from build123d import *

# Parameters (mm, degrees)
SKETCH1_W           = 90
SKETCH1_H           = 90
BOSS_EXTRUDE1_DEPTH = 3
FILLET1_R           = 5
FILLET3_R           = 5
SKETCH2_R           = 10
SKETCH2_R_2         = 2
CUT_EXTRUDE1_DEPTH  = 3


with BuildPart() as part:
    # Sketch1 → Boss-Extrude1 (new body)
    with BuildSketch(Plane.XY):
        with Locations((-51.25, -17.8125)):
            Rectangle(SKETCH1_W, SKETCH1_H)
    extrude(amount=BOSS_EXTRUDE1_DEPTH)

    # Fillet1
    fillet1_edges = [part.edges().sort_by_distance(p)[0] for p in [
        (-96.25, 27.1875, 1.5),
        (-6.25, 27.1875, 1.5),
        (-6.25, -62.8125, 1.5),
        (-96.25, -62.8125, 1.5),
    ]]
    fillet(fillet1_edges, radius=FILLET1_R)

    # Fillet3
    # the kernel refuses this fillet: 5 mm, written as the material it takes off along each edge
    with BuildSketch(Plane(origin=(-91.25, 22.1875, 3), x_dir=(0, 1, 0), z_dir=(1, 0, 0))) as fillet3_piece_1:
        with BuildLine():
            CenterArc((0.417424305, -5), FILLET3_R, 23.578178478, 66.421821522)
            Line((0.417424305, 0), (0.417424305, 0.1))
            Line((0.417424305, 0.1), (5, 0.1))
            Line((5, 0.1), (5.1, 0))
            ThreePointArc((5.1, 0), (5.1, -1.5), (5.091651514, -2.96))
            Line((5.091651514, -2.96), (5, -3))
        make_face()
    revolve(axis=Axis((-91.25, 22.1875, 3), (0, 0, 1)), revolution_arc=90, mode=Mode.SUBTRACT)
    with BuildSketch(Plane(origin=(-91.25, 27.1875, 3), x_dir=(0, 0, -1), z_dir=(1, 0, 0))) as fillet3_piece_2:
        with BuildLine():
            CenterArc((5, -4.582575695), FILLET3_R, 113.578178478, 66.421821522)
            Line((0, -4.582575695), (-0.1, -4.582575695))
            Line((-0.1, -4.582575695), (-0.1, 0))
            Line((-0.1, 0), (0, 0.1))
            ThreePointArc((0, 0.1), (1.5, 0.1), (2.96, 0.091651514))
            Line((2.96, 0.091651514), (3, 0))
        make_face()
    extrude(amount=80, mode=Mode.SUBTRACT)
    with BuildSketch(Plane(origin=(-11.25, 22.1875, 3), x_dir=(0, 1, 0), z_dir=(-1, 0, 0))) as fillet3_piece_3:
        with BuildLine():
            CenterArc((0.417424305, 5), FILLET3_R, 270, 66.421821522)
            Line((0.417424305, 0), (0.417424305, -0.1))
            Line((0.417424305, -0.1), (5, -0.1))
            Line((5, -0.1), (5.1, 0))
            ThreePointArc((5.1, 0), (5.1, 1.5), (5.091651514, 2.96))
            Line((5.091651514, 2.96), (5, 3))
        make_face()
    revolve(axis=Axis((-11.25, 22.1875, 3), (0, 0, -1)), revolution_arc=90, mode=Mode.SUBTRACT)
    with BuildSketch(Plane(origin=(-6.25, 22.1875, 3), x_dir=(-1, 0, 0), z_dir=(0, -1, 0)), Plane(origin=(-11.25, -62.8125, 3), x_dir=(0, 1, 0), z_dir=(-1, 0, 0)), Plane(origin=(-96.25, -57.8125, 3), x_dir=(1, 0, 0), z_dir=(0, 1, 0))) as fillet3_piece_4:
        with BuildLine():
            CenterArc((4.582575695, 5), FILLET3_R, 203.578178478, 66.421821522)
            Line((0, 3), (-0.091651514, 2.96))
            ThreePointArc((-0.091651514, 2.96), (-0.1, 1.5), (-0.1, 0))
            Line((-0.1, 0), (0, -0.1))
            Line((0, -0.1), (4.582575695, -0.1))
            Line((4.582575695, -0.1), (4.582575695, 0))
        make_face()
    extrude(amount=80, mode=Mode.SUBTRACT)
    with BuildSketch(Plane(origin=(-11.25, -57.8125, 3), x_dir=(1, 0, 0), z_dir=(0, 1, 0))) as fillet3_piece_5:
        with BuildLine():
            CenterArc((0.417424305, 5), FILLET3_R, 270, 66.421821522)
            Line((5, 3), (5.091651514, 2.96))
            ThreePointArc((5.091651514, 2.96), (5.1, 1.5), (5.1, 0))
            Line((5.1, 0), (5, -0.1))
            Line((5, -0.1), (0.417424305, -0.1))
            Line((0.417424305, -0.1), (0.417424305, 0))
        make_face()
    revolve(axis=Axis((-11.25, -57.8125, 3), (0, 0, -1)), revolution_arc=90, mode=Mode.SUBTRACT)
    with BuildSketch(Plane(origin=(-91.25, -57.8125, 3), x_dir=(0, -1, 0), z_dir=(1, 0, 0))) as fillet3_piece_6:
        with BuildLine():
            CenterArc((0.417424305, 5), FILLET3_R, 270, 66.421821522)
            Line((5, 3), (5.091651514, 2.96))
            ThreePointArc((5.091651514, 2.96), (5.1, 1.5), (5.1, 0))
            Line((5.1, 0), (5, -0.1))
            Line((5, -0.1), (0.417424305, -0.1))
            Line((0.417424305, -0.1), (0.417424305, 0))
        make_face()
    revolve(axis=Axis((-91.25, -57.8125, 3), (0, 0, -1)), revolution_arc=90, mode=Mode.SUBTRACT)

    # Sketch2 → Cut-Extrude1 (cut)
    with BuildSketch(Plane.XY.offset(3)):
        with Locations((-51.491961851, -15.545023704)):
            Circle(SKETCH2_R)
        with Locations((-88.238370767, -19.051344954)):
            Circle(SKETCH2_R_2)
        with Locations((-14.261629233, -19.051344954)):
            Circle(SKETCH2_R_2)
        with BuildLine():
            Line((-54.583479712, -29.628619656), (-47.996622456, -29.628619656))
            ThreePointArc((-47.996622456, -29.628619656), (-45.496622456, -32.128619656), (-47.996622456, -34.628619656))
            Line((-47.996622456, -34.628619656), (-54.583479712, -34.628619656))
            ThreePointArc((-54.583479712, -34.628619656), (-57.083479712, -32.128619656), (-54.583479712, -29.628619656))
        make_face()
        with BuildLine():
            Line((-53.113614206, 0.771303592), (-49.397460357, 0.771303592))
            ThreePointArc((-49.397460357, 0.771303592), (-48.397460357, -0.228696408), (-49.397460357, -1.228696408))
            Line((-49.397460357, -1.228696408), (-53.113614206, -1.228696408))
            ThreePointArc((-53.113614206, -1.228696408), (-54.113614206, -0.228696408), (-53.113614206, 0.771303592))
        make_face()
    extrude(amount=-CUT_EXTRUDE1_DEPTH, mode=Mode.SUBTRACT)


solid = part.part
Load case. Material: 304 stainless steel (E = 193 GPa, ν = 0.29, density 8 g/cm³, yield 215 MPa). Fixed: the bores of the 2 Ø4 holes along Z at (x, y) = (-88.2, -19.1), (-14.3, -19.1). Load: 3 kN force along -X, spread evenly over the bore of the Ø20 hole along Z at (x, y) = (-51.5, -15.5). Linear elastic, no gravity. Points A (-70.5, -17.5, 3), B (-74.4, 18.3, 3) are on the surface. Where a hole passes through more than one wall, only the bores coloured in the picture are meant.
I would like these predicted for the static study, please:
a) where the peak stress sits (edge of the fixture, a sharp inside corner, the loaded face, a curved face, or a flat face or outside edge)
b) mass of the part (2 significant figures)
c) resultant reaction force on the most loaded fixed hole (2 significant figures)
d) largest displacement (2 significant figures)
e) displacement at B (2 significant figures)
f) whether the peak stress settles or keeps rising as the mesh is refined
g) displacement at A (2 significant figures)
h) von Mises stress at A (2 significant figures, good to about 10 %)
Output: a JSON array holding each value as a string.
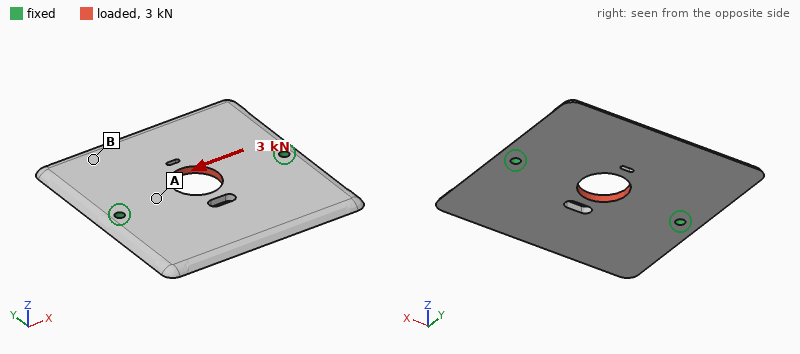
["edge of the fixture", "170 g", "1.5 kN", "4.5 µm", "3.3 µm", "keeps rising", "2.5 µm", "21 MPa"]
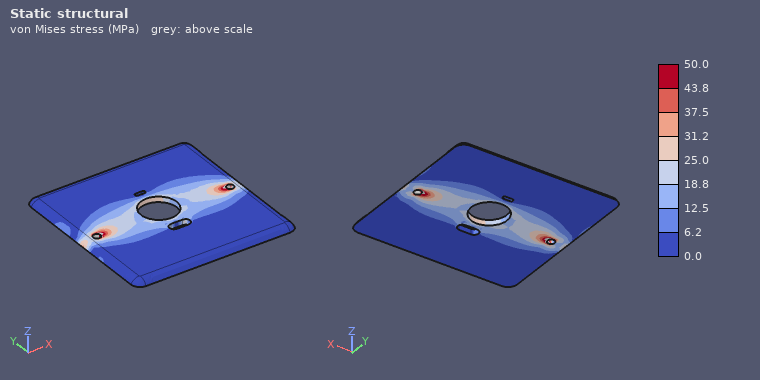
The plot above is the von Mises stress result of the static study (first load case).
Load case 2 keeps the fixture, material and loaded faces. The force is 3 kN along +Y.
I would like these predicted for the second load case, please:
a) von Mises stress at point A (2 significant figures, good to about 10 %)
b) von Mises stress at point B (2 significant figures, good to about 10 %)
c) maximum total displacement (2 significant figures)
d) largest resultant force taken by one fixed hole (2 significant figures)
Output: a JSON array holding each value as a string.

["14 MPa", "6.9 MPa", "7.0 µm", "1.5 kN"]
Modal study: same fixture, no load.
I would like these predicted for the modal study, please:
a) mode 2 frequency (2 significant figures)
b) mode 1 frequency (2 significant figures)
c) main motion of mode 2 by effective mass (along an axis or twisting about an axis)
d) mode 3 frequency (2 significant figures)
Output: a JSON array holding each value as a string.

["1100 Hz", "800 Hz", "along Z", "1800 Hz"]
